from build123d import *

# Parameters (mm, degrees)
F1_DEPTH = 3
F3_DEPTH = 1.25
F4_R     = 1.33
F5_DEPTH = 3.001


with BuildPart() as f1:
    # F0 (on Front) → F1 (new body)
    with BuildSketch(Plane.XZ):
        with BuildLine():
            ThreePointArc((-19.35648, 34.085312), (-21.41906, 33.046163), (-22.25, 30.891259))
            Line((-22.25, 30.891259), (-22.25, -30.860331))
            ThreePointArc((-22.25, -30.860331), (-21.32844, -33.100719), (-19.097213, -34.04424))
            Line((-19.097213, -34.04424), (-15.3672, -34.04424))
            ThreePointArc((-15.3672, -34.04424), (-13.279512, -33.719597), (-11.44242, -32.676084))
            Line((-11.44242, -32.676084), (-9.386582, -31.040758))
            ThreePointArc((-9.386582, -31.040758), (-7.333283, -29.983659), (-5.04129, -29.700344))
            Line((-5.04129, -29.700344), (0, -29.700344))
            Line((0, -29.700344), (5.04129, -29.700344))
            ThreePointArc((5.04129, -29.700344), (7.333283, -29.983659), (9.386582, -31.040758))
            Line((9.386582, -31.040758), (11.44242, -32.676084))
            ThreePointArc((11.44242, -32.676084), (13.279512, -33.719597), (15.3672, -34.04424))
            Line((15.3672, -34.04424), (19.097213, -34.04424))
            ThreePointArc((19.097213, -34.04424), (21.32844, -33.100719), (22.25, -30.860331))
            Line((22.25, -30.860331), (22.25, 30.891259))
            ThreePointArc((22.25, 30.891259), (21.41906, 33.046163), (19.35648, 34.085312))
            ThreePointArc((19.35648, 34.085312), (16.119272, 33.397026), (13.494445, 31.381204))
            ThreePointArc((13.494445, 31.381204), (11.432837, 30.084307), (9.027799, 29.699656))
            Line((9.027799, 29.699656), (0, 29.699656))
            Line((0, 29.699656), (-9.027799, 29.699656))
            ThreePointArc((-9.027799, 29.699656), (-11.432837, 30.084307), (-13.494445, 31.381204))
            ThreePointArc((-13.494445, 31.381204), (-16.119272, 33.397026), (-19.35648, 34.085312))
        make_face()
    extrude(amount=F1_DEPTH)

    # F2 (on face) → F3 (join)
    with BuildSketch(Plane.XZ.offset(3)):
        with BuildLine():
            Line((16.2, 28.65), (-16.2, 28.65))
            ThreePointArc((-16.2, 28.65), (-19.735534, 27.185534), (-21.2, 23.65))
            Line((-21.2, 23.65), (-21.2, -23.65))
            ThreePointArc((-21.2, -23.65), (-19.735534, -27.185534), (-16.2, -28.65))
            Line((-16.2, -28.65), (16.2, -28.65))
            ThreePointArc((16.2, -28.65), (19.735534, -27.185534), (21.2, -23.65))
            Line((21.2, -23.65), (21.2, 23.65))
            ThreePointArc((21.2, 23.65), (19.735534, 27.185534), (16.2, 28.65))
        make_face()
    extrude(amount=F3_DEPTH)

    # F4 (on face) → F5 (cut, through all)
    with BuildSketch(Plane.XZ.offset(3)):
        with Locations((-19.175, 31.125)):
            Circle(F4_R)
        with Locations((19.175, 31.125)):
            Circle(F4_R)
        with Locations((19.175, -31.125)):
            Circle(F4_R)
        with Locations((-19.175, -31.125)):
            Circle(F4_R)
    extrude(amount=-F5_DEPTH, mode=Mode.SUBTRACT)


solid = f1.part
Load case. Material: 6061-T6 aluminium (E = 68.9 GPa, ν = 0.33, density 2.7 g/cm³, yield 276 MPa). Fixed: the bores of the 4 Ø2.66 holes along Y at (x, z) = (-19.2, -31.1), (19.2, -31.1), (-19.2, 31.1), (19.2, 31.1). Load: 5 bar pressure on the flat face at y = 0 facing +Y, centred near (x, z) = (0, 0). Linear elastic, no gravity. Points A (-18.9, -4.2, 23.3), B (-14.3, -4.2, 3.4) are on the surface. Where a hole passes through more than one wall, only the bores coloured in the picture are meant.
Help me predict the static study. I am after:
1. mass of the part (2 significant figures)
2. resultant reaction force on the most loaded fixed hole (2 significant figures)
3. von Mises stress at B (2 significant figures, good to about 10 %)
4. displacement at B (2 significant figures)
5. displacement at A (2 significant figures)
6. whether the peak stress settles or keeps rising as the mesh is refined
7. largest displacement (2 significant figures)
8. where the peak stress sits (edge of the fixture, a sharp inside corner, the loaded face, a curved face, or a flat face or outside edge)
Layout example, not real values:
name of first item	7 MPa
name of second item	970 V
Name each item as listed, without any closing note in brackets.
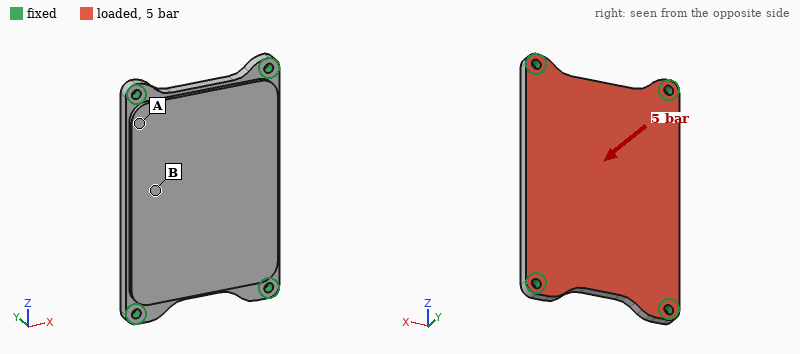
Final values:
mass of the part	31 g
resultant reaction force on the most loaded fixed hole	490 N
von Mises stress at B	46 MPa
displacement at B	0.10 mm
displacement at A	0.031 mm
whether the peak stress settles or keeps rising as the mesh is refined	keeps rising
largest displacement	0.10 mm
where the peak stress sits	edge of the fixture
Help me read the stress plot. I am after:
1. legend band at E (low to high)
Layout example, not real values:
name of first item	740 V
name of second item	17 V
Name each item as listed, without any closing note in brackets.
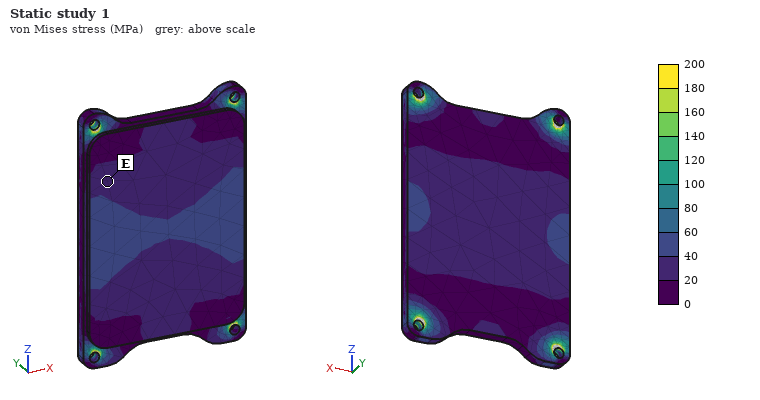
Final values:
legend band at E	20 to 40 MPa
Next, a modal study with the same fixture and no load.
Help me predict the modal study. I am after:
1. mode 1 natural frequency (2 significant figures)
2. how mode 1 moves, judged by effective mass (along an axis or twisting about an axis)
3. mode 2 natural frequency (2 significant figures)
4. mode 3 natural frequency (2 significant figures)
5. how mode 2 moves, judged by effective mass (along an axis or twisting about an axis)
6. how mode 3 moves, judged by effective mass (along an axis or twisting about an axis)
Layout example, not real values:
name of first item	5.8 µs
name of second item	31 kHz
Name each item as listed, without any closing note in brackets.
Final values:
mode 1 natural frequency	3700 Hz
how mode 1 moves, judged by effective mass	along Y
mode 2 natural frequency	6500 Hz
mode 3 natural frequency	9800 Hz
how mode 2 moves, judged by effective mass	twisting about Z
how mode 3 moves, judged by effective mass	twisting about X
